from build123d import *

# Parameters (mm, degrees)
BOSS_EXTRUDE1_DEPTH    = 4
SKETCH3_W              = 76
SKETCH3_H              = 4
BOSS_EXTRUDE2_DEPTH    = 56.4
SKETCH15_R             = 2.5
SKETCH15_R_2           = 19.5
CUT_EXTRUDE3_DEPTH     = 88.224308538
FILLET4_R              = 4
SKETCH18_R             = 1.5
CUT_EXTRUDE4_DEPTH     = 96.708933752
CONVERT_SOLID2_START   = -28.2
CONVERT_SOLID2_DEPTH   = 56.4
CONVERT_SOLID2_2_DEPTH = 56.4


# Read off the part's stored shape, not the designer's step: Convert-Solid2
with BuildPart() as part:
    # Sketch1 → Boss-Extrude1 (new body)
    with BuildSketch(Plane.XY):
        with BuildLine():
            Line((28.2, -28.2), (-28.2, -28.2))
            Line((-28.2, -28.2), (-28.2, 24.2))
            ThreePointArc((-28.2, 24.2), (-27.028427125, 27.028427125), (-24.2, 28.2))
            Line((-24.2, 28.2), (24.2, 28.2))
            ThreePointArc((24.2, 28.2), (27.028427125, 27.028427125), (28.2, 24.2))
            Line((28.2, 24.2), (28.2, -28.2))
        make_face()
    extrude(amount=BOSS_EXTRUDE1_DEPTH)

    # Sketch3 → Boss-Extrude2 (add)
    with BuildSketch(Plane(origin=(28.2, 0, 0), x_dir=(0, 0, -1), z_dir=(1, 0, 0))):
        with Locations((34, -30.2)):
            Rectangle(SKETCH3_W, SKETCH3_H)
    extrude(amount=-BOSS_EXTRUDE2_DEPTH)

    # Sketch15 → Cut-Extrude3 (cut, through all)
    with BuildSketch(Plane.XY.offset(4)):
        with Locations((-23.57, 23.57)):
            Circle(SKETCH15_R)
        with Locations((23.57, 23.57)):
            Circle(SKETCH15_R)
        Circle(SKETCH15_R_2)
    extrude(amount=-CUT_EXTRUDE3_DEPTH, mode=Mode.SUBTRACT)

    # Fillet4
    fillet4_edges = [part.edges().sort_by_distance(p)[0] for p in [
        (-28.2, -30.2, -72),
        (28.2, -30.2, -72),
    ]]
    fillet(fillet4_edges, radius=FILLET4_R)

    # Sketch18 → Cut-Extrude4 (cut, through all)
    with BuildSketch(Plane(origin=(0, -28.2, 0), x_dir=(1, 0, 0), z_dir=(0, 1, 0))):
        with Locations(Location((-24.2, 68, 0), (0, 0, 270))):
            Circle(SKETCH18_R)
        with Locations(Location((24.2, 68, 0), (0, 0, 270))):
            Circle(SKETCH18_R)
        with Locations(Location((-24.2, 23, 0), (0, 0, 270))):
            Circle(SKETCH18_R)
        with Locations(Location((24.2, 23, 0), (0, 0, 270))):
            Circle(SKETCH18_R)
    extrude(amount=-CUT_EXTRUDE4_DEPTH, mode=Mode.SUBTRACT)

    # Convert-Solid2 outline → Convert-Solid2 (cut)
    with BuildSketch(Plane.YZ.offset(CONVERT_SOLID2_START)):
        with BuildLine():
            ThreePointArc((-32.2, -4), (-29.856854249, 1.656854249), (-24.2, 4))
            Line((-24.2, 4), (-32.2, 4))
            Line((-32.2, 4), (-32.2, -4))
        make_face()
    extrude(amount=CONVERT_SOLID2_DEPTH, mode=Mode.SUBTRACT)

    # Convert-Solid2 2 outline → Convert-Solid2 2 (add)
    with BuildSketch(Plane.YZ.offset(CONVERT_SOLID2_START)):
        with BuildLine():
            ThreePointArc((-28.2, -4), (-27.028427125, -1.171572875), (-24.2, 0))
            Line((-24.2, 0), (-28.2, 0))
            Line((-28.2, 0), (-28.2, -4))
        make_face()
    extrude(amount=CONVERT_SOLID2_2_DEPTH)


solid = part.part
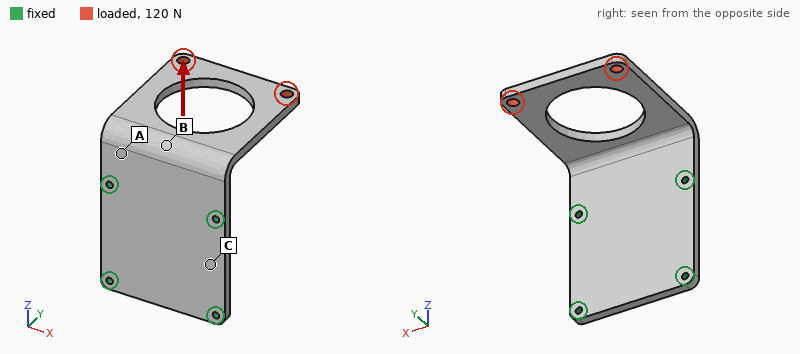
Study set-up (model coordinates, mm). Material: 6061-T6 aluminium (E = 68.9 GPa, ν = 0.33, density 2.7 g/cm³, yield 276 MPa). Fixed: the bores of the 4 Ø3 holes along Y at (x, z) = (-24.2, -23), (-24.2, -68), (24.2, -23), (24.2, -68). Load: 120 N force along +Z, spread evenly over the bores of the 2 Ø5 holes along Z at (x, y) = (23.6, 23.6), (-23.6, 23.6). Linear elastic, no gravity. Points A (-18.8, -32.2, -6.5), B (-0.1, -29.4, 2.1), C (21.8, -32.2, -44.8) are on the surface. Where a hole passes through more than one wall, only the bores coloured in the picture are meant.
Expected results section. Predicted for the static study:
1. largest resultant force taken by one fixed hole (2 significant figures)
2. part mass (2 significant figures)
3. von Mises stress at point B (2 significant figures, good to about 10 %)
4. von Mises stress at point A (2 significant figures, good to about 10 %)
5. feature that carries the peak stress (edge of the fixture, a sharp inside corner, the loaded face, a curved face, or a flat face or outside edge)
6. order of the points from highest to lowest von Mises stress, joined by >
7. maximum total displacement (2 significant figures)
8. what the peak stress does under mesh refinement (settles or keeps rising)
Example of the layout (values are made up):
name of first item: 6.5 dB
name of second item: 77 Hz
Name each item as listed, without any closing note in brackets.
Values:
largest resultant force taken by one fixed hole: 50 N
part mass: 65 g
von Mises stress at point B: 22 MPa
von Mises stress at point A: 39 MPa
feature that carries the peak stress: edge of the fixture
order of the points from highest to lowest von Mises stress, joined by >: A > B > C
maximum total displacement: 1.1 mm
what the peak stress does under mesh refinement: keeps rising
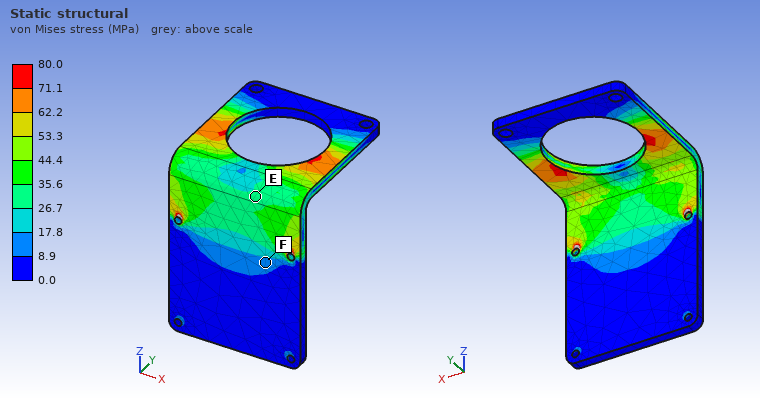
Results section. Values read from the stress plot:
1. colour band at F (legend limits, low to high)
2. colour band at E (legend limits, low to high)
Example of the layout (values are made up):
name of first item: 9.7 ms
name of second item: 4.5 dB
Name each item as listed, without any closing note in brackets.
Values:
colour band at F: 8.9 to 17.8 MPa
colour band at E: 26.7 to 35.6 MPa
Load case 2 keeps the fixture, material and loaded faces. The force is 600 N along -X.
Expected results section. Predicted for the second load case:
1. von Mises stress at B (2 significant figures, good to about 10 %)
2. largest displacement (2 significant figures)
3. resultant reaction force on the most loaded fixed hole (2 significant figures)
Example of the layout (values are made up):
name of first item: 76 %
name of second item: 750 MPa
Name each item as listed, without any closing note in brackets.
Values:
von Mises stress at B: 56 MPa
largest displacement: 0.76 mm
resultant reaction force on the most loaded fixed hole: 830 N
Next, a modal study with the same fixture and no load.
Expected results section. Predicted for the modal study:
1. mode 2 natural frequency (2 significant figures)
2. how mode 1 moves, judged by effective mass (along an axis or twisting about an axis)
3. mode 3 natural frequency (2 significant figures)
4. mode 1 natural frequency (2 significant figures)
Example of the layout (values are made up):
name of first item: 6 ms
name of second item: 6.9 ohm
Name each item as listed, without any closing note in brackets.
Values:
mode 2 natural frequency: 1400 Hz
how mode 1 moves, judged by effective mass: along Z
mode 3 natural frequency: 2000 Hz
mode 1 natural frequency: 610 Hz
